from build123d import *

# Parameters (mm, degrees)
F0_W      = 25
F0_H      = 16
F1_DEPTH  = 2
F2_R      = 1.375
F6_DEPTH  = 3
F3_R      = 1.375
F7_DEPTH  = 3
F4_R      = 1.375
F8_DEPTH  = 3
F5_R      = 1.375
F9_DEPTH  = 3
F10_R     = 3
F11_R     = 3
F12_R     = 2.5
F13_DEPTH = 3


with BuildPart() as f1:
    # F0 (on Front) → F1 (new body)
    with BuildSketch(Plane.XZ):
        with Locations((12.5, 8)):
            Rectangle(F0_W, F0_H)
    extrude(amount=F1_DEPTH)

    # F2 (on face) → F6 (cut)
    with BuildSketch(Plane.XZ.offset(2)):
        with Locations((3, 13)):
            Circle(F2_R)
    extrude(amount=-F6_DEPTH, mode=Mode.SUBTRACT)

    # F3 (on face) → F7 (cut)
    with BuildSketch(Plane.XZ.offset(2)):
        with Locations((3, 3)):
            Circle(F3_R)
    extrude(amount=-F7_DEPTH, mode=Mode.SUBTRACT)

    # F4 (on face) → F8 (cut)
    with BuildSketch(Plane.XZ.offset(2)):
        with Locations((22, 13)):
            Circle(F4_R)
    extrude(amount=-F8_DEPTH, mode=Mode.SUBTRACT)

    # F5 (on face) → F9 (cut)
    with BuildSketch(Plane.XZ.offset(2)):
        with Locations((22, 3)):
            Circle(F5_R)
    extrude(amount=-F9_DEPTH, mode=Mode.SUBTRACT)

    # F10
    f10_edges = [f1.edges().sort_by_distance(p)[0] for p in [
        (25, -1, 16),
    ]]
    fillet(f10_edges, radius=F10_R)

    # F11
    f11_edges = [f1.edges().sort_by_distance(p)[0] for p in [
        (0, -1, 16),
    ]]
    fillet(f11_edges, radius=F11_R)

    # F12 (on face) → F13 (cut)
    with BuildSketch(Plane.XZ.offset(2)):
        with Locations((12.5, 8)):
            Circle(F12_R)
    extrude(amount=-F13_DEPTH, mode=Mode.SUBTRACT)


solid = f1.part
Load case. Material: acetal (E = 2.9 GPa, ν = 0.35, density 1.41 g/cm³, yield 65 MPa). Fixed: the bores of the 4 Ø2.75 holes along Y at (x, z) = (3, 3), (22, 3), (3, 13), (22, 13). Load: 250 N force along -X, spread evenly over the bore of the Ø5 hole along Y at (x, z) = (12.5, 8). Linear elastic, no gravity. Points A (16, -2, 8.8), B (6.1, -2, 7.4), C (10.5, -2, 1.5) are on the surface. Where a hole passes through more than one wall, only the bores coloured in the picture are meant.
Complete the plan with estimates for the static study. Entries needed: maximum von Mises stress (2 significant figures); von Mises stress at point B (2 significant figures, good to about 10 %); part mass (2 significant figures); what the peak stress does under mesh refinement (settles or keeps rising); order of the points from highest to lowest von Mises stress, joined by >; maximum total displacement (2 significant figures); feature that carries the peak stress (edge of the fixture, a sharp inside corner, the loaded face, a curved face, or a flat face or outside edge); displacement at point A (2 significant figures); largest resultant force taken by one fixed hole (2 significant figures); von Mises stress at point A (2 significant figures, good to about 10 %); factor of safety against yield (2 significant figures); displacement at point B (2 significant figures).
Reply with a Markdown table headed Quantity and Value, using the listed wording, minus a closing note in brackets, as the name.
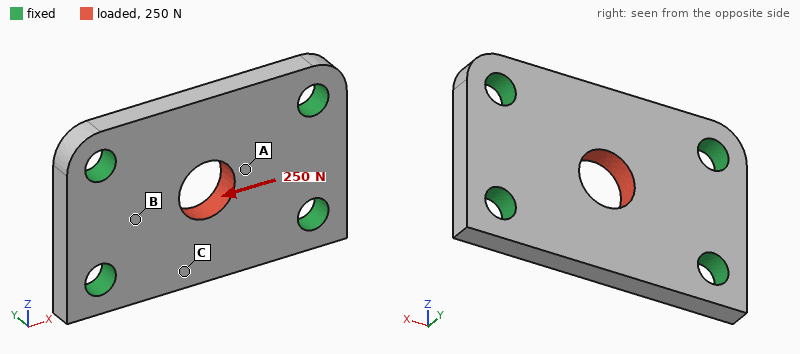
| Quantity | Value |
|---|---|
| maximum von Mises stress | 14 MPa |
| von Mises stress at point B | 4.2 MPa |
| part mass | 0.99 g |
| what the peak stress does under mesh refinement | settles |
| order of the points from highest to lowest von Mises stress, joined by > | A > B > C |
| maximum total displacement | 18 µm |
| feature that carries the peak stress | the loaded face |
| displacement at point A | 15 µm |
| largest resultant force taken by one fixed hole | 66 N |
| von Mises stress at point A | 7.5 MPa |
| factor of safety against yield | 4.8 |
| displacement at point B | 8.7 µm |
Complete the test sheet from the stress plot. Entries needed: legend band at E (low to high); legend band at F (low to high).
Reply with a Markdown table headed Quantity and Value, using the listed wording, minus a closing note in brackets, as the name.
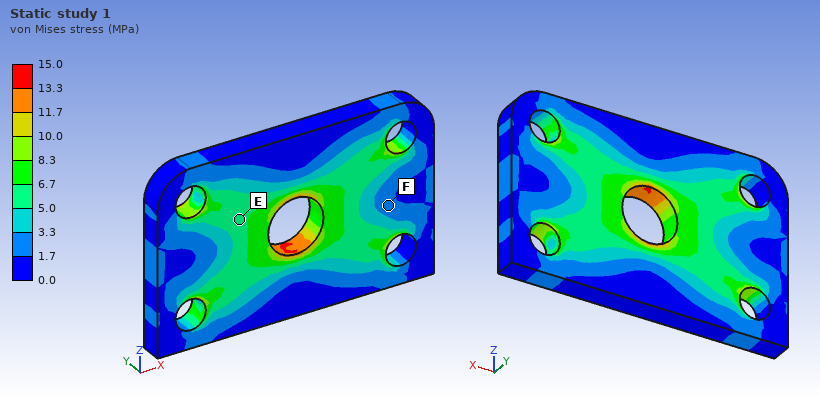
| Quantity | Value |
|---|---|
| legend band at E | 5.0 to 6.7 MPa |
| legend band at F | 1.7 to 3.3 MPa |
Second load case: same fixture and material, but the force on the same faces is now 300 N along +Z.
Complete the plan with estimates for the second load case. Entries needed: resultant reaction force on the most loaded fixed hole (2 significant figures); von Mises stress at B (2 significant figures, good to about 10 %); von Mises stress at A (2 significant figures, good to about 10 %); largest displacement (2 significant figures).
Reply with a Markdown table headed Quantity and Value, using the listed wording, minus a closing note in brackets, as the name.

| Quantity | Value |
|---|---|
| resultant reaction force on the most loaded fixed hole | 92 N |
| von Mises stress at B | 10 MPa |
| von Mises stress at A | 13 MPa |
| largest displacement | 48 µm |
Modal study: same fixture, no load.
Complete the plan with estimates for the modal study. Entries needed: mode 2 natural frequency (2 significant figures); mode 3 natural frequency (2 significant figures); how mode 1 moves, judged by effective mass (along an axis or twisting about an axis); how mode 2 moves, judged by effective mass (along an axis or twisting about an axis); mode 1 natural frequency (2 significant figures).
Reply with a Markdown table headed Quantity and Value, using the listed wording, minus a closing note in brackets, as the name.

| Quantity | Value |
|---|---|
| mode 2 natural frequency | 11 kHz |
| mode 3 natural frequency | 17 kHz |
| how mode 1 moves, judged by effective mass | along Y |
| how mode 2 moves, judged by effective mass | twisting about X |
| mode 1 natural frequency | 9000 Hz |
